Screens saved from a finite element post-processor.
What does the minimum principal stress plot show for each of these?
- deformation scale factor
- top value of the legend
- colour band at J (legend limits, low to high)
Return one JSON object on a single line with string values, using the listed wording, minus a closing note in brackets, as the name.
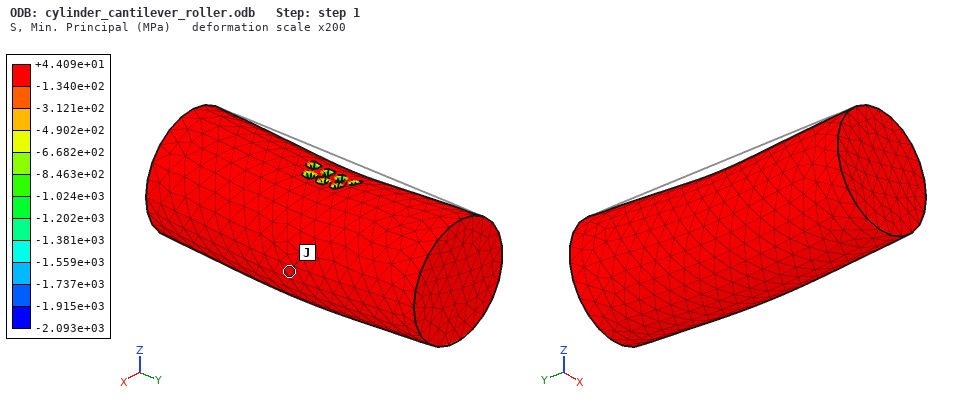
{"deformation scale factor": "200", "top value of the legend": "+4.409e+01 MPa", "colour band at J": "-1.340e+02 to +4.409e+01 MPa"}
